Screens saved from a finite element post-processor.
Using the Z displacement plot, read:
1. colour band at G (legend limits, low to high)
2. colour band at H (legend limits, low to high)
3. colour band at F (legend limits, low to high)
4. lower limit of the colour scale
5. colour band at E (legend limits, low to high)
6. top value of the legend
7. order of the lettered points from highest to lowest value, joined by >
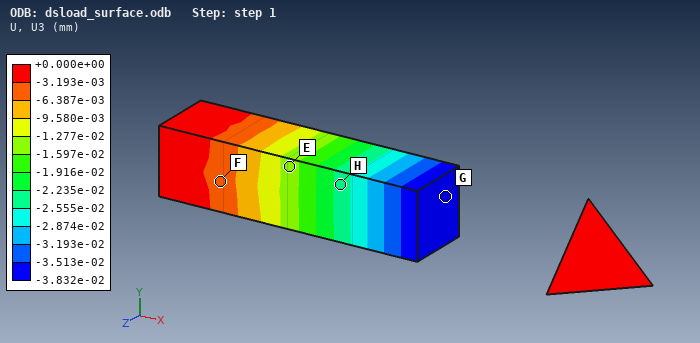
-3.832e-02 to -3.513e-02 mm
-2.555e-02 to -2.235e-02 mm
-6.387e-03 to -3.193e-03 mm
-3.832e-02 mm
-1.597e-02 to -1.277e-02 mm
+0.000e+00 mm
F > E > H > G
